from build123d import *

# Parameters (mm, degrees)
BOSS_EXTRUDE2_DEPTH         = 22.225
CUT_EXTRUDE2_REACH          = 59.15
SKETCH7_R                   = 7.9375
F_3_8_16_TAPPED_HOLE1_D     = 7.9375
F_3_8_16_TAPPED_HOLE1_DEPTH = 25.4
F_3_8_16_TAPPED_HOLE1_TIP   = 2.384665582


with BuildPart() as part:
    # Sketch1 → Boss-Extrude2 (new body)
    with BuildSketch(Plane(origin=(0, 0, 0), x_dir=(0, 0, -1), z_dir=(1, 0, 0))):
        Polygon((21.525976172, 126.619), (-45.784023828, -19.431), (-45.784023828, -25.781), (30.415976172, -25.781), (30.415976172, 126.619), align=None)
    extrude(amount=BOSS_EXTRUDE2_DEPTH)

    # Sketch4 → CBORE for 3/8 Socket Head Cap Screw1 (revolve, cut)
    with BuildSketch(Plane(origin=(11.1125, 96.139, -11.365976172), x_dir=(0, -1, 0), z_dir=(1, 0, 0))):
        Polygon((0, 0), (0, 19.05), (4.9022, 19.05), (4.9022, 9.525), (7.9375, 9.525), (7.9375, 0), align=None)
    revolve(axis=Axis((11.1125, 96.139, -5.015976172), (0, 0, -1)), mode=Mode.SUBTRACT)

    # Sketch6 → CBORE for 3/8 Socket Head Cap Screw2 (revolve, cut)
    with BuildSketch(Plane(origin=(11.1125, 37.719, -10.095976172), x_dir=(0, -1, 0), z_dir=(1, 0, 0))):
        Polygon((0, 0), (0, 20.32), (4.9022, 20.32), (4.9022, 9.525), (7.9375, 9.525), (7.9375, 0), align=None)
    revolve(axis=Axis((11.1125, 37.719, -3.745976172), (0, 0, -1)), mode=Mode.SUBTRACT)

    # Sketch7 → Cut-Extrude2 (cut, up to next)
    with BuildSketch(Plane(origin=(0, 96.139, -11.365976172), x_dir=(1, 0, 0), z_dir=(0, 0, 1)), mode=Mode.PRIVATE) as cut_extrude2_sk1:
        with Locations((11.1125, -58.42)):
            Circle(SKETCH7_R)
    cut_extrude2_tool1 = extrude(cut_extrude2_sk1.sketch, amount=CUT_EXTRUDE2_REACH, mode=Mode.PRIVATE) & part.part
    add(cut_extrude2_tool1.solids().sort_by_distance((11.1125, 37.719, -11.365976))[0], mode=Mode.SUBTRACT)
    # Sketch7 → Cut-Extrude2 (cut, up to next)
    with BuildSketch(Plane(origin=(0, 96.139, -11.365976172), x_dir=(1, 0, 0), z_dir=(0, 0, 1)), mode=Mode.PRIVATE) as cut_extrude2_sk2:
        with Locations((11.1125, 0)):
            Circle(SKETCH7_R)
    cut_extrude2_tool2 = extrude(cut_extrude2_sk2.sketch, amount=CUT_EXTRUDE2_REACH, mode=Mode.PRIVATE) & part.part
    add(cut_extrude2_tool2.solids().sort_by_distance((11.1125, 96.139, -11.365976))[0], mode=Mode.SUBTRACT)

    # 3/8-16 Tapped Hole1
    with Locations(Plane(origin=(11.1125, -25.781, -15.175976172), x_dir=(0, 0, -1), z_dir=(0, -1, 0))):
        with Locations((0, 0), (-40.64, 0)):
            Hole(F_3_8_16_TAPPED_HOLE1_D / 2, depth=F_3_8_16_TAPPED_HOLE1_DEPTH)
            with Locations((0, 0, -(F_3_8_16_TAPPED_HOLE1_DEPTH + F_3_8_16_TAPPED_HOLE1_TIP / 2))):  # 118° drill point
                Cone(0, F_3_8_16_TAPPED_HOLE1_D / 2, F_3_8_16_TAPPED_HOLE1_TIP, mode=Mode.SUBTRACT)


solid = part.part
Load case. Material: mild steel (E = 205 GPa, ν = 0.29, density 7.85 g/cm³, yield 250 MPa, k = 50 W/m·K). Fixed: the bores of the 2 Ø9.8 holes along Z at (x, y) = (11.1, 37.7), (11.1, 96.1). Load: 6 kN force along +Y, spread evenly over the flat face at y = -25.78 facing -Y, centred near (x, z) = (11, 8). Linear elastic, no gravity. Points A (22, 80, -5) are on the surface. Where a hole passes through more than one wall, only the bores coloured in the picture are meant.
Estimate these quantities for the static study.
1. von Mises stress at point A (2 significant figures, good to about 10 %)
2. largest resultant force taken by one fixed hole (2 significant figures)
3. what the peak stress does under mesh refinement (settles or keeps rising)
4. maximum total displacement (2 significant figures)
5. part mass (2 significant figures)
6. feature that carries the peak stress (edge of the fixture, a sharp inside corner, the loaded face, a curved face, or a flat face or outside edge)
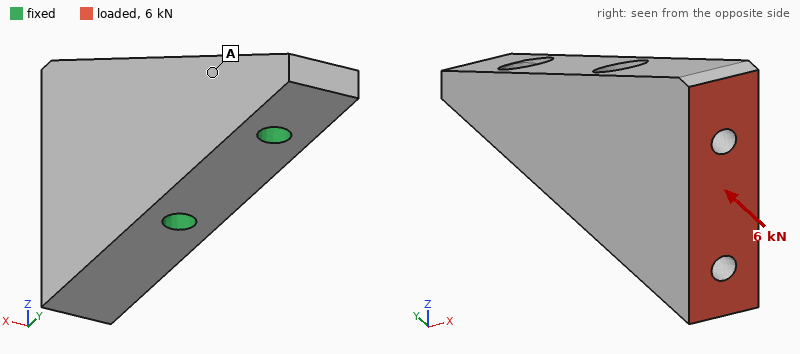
12 MPa
4.5 kN
keeps rising
25 µm
1.1 kg
edge of the fixture
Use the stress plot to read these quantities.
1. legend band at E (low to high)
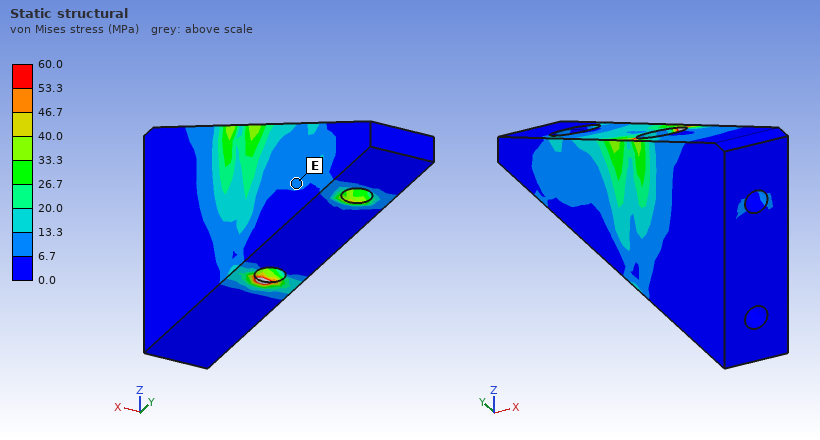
6.7 to 13.3 MPa
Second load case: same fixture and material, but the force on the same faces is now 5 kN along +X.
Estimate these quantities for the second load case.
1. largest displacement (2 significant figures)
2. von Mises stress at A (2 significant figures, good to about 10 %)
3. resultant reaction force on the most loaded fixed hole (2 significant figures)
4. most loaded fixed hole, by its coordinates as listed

0.17 mm
29 MPa
8.2 kN
(11.1, 37.7)
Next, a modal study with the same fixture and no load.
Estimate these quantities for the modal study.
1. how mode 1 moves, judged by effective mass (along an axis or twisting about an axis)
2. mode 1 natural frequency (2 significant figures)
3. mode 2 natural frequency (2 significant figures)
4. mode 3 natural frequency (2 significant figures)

along X
1800 Hz
3100 Hz
4200 Hz
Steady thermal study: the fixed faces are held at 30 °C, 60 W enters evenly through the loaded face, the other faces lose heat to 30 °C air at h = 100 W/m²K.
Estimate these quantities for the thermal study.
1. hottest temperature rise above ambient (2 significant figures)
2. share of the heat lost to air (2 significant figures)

49 K
66 %
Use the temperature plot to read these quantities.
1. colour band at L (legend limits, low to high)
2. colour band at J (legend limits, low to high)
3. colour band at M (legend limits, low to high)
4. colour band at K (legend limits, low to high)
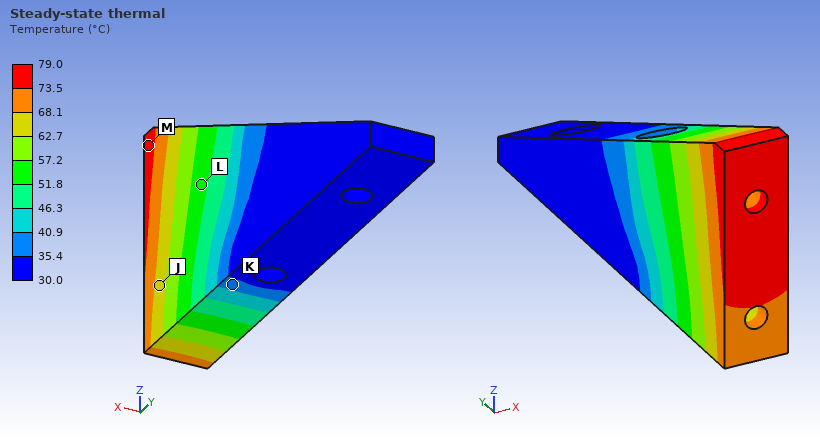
51.8 to 57.2 °C
62.7 to 68.1 °C
73.5 to 79.0 °C
35.4 to 40.9 °C
